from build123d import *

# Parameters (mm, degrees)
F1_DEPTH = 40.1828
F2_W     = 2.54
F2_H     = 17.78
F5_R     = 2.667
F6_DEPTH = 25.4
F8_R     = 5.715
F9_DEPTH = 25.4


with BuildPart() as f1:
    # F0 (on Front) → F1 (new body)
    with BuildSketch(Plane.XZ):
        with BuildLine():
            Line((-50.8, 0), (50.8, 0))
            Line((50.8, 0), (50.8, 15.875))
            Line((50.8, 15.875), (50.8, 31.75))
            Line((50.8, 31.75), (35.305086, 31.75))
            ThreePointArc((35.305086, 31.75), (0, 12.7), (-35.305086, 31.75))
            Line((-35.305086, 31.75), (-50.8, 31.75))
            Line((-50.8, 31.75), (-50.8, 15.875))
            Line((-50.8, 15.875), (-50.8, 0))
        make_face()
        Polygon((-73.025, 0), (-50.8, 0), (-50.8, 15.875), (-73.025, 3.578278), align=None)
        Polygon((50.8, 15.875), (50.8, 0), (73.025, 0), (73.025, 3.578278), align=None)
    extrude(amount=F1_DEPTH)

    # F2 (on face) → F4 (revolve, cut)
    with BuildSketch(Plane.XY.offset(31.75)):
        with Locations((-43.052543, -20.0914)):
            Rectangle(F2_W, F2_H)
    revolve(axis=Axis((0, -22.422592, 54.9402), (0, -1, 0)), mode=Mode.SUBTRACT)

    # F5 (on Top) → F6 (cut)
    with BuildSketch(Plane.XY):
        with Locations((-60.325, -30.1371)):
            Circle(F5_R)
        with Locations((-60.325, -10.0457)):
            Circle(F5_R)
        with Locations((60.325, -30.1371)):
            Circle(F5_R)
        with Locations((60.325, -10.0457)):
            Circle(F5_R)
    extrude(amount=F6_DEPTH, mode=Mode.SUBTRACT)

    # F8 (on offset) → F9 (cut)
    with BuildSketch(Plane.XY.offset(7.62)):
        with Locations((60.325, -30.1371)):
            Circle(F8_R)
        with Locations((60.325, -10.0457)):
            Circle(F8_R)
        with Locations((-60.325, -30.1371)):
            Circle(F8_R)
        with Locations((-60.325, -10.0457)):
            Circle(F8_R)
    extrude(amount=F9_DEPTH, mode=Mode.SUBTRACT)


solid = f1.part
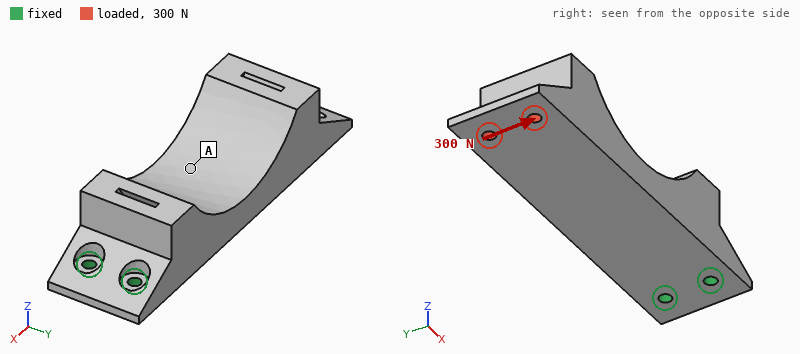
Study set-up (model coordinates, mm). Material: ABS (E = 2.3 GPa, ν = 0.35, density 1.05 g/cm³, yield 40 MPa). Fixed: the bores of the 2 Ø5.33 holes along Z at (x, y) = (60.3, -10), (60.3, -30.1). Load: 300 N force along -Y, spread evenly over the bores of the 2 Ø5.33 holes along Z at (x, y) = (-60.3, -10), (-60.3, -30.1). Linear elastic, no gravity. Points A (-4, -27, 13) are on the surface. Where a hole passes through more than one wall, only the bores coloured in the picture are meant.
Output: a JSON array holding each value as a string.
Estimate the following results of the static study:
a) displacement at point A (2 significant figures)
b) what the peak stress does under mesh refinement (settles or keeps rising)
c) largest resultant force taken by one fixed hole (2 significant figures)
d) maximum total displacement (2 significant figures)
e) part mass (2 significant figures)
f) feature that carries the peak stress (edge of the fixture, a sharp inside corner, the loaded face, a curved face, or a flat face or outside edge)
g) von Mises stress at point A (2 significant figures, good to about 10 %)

["0.60 mm", "keeps rising", "1.6 kN", "1.7 mm", "110 g", "edge of the fixture", "2.4 MPa"]
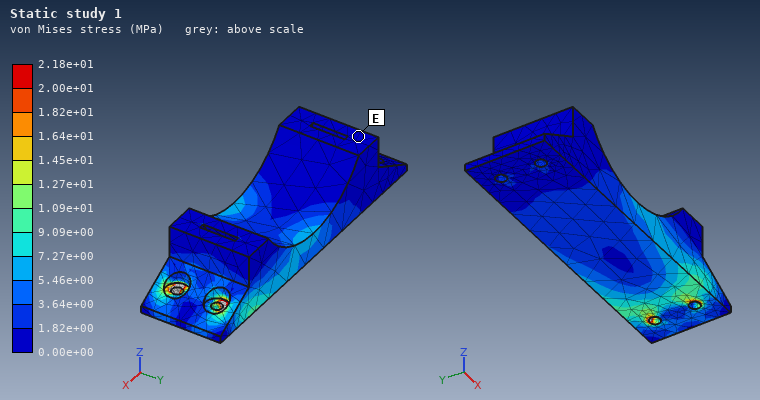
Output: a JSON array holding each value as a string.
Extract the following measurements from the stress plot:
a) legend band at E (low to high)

["0.00e+00 to 1.82e+00 MPa"]
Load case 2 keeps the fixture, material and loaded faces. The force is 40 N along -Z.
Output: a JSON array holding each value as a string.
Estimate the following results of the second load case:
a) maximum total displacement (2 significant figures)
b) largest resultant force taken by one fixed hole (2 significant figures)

["1.6 mm", "21 N"]
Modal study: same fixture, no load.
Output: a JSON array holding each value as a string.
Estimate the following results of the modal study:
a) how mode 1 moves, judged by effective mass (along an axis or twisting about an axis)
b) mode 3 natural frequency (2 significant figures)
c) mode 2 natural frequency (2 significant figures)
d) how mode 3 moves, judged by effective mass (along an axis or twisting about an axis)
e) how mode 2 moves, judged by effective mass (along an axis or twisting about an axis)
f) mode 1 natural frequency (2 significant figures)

["along Z", "950 Hz", "400 Hz", "twisting about X", "along Y", "150 Hz"]
